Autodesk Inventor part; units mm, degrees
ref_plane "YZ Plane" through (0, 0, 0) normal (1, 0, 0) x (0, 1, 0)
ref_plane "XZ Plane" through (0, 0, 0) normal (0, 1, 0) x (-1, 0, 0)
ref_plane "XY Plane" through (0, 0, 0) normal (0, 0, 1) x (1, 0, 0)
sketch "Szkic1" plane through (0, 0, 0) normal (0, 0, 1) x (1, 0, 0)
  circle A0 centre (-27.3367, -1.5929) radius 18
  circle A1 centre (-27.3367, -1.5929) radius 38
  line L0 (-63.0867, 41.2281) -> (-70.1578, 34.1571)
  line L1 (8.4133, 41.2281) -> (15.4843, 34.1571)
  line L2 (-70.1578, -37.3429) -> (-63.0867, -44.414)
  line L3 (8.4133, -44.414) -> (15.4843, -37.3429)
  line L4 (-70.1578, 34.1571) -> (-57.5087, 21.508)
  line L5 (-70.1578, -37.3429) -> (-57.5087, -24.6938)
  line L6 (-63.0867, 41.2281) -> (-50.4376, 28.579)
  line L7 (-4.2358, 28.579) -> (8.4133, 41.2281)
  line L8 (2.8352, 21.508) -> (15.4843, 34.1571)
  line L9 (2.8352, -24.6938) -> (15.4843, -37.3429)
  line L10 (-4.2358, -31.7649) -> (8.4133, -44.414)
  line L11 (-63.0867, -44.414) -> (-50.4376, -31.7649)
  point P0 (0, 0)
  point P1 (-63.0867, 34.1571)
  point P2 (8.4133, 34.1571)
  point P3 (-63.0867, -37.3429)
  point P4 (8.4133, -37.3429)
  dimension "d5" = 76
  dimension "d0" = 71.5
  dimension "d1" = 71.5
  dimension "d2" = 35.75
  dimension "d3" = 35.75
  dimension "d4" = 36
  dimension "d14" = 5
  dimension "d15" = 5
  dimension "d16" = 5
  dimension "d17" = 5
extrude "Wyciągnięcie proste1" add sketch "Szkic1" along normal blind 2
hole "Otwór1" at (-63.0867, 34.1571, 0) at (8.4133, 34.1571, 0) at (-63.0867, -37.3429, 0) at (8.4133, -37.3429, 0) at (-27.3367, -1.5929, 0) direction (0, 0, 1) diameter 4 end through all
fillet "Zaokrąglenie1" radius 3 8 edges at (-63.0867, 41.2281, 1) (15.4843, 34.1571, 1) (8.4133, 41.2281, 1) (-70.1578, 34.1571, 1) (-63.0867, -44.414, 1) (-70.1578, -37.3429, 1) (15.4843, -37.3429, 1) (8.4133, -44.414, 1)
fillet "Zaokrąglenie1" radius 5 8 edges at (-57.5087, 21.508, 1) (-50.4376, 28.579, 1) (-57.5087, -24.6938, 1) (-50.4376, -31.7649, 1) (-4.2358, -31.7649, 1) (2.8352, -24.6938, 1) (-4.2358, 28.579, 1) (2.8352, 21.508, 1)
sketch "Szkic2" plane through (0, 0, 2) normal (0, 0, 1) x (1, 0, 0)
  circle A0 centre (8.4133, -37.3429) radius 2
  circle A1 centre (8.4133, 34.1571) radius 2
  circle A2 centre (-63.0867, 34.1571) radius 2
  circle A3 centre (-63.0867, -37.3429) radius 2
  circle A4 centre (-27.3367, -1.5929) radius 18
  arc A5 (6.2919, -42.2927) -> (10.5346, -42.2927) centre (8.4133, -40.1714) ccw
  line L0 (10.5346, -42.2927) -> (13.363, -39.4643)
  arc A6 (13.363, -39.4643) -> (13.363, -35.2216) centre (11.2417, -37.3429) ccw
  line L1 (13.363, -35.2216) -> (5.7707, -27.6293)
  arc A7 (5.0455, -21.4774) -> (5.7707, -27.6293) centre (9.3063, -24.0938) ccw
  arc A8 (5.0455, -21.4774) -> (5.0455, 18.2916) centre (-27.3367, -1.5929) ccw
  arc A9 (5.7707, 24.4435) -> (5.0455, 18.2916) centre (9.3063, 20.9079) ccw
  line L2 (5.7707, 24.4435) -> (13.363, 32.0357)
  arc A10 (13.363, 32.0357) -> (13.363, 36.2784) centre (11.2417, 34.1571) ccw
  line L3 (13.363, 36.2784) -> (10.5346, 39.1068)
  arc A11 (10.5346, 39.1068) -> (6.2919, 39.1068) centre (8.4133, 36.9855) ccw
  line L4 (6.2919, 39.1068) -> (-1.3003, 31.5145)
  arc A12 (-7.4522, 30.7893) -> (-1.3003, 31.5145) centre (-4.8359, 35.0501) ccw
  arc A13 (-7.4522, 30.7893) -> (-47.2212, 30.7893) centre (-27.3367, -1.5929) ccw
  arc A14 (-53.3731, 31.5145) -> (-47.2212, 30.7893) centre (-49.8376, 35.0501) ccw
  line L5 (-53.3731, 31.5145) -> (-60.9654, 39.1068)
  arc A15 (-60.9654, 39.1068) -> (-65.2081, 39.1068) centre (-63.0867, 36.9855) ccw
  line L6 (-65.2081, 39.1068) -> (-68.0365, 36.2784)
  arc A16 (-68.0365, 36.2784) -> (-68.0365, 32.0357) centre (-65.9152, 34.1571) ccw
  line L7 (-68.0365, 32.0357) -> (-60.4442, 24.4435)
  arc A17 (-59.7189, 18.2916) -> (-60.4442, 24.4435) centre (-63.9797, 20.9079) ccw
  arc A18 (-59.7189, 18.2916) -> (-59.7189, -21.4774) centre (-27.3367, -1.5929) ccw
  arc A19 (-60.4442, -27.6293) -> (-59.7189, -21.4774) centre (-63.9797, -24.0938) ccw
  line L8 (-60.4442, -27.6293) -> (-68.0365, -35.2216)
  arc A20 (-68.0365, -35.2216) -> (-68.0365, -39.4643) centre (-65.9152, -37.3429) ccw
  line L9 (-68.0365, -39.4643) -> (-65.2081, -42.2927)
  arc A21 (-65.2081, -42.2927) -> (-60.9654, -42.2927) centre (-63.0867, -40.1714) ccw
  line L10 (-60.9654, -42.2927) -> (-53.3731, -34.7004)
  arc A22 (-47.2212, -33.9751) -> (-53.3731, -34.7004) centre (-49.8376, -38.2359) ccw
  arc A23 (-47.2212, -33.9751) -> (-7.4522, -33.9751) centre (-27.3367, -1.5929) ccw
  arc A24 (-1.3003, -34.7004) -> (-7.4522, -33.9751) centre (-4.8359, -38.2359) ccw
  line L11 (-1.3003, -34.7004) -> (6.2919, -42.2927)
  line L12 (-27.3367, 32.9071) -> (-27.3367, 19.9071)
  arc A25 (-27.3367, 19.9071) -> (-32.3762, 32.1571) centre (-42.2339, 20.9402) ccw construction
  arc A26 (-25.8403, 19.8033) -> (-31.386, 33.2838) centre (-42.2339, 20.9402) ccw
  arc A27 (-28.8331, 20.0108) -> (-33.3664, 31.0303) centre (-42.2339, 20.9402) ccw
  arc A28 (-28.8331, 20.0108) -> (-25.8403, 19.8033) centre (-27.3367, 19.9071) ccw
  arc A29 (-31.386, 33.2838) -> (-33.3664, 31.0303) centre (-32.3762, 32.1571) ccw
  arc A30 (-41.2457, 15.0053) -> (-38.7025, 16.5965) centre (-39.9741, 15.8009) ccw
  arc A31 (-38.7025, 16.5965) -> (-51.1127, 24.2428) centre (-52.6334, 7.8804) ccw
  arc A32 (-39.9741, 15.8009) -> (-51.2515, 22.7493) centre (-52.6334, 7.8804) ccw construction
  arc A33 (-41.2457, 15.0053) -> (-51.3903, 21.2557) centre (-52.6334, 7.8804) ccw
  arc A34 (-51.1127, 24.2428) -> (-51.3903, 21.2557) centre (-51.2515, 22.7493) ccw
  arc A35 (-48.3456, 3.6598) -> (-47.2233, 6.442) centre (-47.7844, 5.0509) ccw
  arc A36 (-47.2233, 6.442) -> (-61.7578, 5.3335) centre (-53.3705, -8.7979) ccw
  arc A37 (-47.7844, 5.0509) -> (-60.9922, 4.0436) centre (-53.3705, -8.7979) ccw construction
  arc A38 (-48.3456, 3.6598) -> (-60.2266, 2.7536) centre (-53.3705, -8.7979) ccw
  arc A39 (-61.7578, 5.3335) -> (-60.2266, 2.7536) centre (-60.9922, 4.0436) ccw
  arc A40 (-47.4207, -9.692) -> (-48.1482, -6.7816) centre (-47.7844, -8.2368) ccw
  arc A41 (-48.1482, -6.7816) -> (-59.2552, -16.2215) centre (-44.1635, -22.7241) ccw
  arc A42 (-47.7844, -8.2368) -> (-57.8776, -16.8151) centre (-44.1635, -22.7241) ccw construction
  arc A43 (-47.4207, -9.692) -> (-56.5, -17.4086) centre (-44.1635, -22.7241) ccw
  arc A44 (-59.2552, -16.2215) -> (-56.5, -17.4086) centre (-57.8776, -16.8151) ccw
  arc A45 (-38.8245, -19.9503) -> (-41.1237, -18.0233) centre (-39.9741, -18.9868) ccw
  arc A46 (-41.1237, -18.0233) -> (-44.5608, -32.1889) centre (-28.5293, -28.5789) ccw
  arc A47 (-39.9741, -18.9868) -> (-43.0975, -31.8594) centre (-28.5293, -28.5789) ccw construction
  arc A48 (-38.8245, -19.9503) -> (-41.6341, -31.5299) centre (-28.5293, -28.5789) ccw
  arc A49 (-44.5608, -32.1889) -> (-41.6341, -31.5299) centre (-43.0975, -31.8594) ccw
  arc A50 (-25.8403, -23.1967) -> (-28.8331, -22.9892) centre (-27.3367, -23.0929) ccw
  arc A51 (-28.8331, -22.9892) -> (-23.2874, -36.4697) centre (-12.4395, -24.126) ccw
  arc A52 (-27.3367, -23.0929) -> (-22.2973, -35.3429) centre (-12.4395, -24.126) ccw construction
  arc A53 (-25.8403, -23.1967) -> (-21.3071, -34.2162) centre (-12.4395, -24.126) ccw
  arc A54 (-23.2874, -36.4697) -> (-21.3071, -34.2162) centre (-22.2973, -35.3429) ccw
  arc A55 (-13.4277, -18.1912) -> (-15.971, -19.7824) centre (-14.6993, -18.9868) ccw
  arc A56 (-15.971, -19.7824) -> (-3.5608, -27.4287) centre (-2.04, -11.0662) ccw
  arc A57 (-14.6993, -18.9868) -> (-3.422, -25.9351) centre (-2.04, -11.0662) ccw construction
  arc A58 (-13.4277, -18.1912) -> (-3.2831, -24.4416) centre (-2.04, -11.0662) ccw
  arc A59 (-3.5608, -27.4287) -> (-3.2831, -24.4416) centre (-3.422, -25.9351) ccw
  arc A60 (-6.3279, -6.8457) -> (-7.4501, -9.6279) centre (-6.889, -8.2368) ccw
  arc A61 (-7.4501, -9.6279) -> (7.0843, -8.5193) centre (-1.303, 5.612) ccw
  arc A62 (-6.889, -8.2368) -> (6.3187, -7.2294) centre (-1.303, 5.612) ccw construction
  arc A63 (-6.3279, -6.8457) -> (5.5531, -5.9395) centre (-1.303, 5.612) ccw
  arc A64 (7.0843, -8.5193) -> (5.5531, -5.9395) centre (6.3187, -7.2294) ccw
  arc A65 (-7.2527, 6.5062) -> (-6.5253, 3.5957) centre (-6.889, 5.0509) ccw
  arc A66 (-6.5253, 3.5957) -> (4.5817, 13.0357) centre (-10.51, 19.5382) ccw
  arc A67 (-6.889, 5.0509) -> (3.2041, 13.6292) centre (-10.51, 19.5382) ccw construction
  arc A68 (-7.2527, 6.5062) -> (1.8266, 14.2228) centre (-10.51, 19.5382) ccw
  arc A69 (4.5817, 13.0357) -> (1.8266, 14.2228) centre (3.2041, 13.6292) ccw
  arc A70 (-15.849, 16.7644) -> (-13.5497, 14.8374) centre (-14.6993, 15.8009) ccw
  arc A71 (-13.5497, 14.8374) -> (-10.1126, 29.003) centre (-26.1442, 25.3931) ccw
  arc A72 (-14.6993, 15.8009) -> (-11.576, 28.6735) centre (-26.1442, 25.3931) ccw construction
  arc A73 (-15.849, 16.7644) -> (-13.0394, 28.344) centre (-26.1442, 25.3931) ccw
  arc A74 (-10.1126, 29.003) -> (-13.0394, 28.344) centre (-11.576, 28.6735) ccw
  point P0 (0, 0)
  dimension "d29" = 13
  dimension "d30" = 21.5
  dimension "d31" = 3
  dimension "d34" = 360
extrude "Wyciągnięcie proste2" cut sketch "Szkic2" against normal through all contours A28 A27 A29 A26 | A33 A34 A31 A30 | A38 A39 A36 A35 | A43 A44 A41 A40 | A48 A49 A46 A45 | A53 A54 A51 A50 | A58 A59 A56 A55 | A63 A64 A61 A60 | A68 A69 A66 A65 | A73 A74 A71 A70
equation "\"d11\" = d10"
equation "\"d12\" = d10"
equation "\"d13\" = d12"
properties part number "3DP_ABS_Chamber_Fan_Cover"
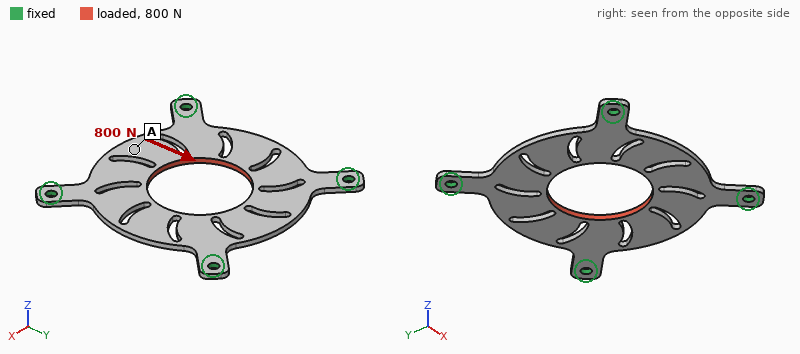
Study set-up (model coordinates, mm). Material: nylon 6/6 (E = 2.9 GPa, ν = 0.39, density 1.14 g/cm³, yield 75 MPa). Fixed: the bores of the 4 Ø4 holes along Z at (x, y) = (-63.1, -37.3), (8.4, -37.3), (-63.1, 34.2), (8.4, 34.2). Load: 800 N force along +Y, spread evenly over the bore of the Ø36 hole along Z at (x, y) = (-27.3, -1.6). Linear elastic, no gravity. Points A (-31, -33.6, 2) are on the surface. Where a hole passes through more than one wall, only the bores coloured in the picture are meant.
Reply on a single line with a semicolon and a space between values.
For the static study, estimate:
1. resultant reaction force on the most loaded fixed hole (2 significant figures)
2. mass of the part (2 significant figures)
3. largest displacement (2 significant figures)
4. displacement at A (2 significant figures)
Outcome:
230 N; 8.4 g; 0.34 mm; 0.33 mm
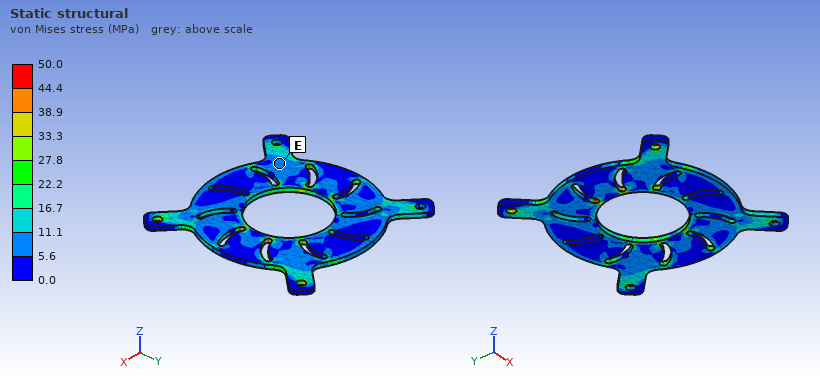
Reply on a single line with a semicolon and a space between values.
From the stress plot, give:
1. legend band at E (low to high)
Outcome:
5.6 to 11.1 MPa
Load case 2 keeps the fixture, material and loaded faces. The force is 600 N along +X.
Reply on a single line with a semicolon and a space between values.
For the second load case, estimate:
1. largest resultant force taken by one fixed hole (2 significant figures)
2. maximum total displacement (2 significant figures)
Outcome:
190 N; 0.26 mm
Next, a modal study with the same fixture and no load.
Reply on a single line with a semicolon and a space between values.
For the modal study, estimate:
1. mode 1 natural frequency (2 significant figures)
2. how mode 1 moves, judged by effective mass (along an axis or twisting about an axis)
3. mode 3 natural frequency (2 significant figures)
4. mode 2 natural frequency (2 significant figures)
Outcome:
380 Hz; along Z; 590 Hz; 590 Hz
